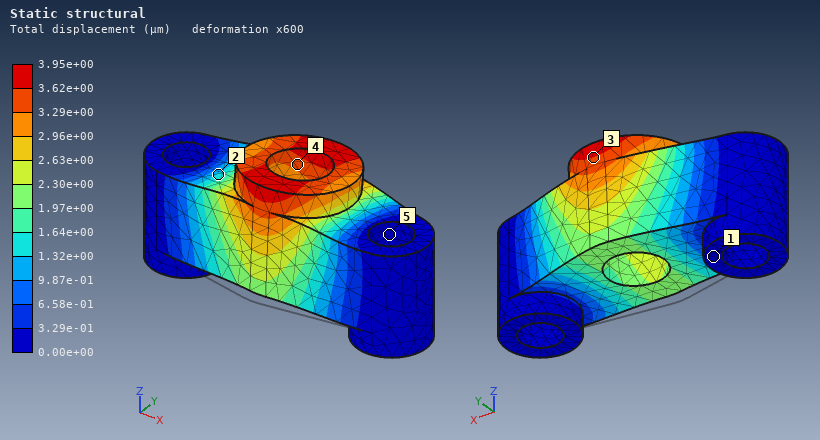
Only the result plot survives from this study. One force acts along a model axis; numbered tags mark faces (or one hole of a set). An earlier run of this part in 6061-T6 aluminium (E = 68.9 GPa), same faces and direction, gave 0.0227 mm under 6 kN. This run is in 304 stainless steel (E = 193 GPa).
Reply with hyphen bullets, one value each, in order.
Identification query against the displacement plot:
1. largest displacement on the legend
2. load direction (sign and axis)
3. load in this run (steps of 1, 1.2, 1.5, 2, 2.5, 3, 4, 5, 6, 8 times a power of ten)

- 3.95e+00 µm
- +Y
- 3 kN
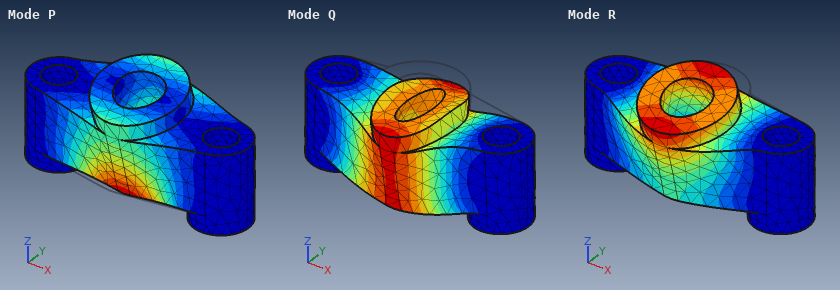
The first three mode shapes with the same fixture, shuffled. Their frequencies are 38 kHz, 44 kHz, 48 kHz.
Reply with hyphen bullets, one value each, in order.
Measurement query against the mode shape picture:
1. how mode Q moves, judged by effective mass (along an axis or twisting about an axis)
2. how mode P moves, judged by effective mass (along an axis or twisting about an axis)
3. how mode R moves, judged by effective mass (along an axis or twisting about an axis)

- along Z
- along Y
- along Y
